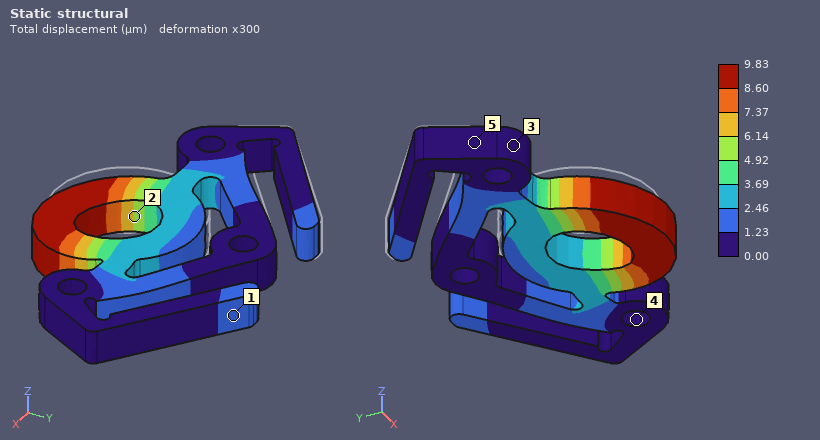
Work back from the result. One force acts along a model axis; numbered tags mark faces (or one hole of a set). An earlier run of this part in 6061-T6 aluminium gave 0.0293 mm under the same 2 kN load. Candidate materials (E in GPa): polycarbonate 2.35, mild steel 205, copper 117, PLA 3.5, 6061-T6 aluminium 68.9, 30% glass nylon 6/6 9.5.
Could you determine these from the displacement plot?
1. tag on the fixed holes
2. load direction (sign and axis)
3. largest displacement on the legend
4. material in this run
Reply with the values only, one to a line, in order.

4
+X
9.83 µm
mild steel
